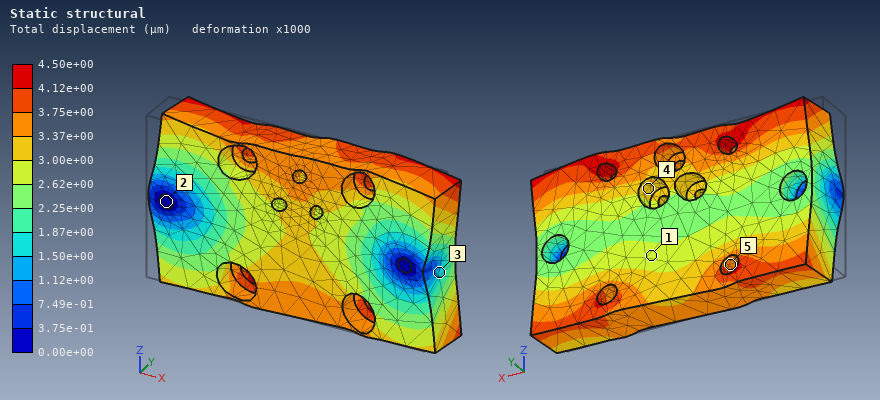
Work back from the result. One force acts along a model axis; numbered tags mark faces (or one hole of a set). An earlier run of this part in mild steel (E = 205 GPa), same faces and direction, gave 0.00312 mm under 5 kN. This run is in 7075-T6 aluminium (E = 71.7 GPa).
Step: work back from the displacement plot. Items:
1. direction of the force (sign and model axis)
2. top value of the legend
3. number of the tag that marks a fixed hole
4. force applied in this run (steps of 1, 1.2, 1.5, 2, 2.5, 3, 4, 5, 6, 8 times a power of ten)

+X
4.50e+00 µm
2
2.5 kN
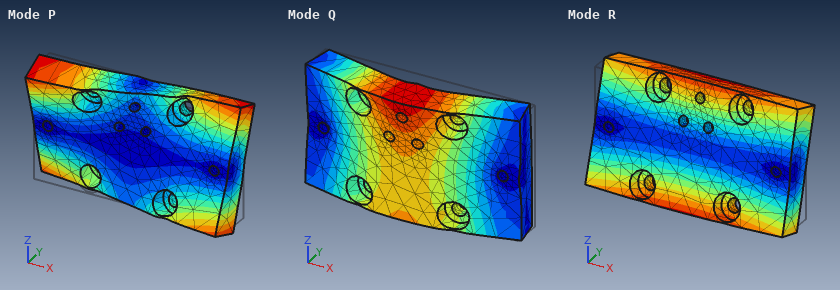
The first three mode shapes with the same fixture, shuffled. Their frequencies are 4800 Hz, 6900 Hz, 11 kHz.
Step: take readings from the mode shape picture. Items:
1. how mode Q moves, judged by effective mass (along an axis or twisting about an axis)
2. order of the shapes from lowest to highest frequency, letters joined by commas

along Y
R, Q, P
